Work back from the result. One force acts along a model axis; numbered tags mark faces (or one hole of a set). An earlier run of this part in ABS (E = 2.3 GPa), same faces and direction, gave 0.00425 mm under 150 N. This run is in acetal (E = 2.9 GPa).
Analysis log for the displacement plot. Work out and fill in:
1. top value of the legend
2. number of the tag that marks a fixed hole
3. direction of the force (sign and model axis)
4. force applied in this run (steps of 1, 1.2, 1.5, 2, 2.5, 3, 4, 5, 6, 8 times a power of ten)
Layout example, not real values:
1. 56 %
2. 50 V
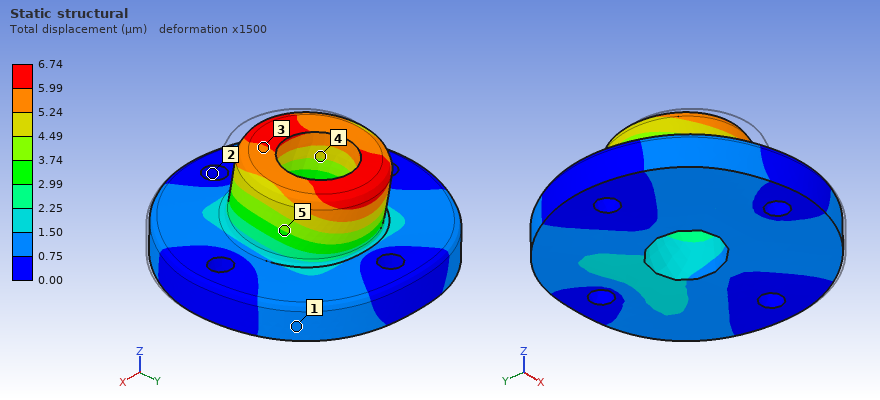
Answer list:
1. 6.74 µm
2. 2
3. +Y
4. 300 N
